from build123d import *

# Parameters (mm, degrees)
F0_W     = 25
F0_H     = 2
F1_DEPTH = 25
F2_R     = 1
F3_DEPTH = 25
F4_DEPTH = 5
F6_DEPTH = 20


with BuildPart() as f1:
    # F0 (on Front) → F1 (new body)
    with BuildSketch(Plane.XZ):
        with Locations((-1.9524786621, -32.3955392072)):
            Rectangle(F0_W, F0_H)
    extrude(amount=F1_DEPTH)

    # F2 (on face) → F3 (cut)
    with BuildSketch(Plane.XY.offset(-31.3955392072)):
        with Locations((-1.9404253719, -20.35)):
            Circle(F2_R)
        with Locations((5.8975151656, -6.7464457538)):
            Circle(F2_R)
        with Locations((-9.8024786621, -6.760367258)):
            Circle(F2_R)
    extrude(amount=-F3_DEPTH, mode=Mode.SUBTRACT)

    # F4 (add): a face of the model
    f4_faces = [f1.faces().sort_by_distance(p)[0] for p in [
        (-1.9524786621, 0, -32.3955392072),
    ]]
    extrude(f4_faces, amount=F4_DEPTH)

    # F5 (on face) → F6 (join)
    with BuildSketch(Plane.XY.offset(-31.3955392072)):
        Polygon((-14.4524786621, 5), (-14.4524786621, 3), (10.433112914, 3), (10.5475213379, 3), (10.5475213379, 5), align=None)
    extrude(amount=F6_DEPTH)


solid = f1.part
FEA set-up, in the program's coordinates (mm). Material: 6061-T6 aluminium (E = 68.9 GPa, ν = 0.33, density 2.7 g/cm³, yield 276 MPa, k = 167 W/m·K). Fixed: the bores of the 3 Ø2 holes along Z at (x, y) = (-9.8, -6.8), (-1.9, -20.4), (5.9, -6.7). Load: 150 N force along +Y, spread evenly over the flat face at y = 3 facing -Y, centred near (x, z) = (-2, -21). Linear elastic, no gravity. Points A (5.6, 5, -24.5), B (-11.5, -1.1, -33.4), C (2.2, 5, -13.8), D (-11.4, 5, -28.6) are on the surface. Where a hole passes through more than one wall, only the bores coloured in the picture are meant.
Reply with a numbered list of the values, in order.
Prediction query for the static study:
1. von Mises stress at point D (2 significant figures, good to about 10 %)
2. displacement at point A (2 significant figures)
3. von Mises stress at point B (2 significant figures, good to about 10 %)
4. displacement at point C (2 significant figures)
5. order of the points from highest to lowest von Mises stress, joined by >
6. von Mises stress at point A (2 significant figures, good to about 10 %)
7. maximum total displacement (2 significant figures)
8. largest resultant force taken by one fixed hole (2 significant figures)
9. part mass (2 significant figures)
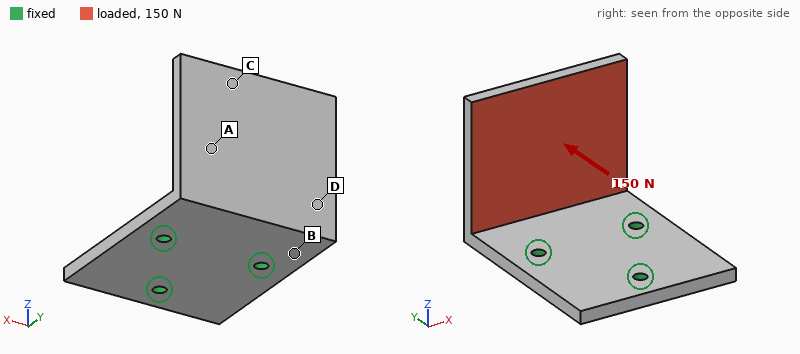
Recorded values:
1. 60 MPa
2. 0.18 mm
3. 90 MPa
4. 0.40 mm
5. B > D > A > C
6. 35 MPa
7. 0.45 mm
8. 69 N
9. 6.7 g
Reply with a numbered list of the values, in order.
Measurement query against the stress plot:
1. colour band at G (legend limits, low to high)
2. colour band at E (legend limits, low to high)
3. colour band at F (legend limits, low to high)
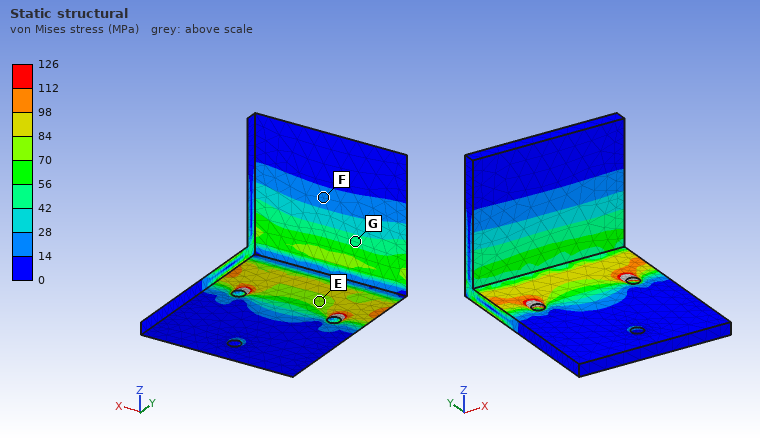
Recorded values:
1. 42 to 56 MPa
2. 70 to 84 MPa
3. 14 to 28 MPa
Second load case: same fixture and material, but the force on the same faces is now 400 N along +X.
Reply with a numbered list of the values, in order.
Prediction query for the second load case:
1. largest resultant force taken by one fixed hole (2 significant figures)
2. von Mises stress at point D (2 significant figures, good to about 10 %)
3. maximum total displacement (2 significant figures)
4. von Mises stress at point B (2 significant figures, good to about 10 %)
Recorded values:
1. 390 N
2. 60 MPa
3. 0.28 mm
4. 86 MPa
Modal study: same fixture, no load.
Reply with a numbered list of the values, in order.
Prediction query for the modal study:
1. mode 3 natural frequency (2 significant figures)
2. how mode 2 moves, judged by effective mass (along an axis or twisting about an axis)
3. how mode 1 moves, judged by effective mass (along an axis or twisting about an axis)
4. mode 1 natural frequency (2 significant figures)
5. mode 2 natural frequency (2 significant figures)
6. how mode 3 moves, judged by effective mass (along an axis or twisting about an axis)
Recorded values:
1. 6800 Hz
2. along X
3. along Y
4. 2100 Hz
5. 4200 Hz
6. along Z
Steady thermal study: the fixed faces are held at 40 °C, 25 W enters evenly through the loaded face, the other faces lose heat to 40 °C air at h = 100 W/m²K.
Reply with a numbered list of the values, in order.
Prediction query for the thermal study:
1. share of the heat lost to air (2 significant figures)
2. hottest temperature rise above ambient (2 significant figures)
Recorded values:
1. 18 %
2. 56 K
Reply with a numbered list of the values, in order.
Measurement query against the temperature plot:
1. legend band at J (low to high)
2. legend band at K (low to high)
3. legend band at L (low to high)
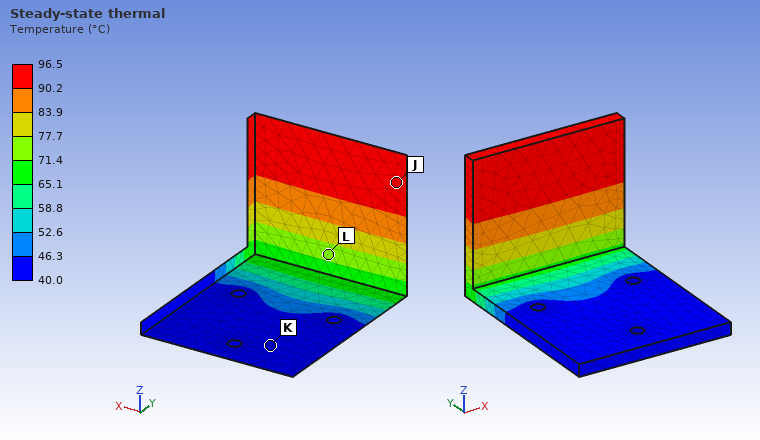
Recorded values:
1. 90.2 to 96.5 °C
2. 40.0 to 46.3 °C
3. 71.4 to 77.7 °C
